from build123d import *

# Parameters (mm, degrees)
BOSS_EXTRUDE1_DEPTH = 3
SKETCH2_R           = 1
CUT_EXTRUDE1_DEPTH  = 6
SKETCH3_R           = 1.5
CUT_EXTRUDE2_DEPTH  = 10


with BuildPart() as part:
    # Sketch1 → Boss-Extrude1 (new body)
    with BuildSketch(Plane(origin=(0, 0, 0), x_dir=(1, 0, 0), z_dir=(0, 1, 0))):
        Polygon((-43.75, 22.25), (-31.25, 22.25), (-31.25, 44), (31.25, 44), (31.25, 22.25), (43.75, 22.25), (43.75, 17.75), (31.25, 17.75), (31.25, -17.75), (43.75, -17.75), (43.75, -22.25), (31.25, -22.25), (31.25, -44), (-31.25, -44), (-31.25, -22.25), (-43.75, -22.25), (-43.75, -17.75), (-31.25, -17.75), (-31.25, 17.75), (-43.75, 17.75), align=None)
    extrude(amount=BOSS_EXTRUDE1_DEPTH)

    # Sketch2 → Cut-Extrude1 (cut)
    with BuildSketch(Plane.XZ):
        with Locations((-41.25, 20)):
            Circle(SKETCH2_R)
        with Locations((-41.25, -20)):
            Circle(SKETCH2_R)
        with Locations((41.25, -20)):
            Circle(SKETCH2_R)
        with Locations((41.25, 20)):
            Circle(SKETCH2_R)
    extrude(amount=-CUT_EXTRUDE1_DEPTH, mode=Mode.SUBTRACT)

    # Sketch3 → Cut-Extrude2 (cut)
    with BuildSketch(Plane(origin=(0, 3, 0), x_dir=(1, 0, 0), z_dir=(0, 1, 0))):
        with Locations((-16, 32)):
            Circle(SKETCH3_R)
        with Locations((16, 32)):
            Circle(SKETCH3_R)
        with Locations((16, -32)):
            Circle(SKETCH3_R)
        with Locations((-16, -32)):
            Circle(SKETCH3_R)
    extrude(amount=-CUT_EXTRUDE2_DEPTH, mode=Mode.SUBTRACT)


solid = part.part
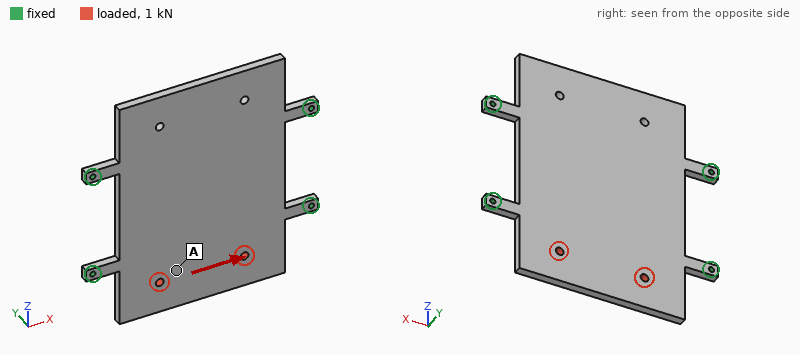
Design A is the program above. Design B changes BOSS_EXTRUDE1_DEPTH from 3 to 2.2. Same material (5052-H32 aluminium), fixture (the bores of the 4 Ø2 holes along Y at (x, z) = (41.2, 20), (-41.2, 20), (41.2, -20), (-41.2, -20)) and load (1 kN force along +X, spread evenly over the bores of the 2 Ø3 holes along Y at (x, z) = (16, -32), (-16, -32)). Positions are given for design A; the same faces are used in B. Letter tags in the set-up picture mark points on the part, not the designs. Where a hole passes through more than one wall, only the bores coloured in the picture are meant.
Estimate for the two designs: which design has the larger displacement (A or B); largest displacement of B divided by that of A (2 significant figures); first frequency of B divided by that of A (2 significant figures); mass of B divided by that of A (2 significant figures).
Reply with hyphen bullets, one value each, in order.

- B
- 1.4
- 0.75
- 0.73
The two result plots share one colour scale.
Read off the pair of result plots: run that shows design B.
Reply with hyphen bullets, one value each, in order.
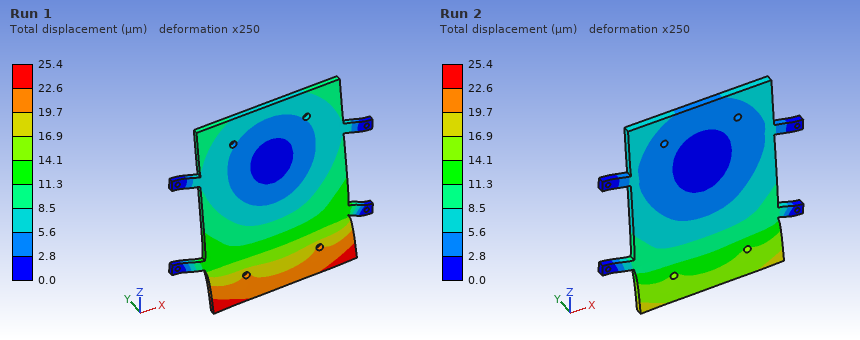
- Run 1
